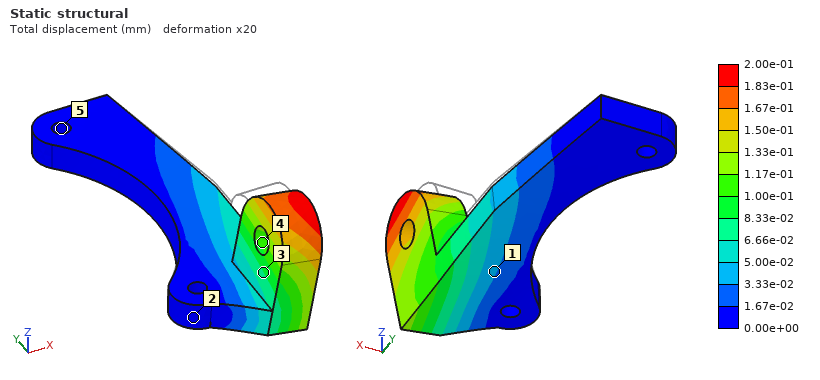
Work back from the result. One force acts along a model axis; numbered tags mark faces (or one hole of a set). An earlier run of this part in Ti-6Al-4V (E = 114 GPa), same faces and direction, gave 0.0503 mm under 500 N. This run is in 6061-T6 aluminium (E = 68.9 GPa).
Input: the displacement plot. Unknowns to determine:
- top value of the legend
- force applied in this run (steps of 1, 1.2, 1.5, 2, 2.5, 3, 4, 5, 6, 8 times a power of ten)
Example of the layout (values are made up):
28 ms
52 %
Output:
2.00e-01 mm
1.2 kN
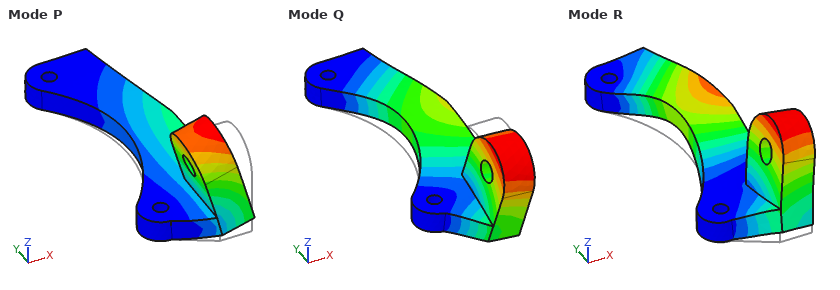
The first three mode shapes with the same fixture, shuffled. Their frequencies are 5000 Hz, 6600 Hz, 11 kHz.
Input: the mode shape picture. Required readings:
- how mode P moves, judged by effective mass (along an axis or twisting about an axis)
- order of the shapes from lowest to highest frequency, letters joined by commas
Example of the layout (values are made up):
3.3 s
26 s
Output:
along Z
P, Q, R
